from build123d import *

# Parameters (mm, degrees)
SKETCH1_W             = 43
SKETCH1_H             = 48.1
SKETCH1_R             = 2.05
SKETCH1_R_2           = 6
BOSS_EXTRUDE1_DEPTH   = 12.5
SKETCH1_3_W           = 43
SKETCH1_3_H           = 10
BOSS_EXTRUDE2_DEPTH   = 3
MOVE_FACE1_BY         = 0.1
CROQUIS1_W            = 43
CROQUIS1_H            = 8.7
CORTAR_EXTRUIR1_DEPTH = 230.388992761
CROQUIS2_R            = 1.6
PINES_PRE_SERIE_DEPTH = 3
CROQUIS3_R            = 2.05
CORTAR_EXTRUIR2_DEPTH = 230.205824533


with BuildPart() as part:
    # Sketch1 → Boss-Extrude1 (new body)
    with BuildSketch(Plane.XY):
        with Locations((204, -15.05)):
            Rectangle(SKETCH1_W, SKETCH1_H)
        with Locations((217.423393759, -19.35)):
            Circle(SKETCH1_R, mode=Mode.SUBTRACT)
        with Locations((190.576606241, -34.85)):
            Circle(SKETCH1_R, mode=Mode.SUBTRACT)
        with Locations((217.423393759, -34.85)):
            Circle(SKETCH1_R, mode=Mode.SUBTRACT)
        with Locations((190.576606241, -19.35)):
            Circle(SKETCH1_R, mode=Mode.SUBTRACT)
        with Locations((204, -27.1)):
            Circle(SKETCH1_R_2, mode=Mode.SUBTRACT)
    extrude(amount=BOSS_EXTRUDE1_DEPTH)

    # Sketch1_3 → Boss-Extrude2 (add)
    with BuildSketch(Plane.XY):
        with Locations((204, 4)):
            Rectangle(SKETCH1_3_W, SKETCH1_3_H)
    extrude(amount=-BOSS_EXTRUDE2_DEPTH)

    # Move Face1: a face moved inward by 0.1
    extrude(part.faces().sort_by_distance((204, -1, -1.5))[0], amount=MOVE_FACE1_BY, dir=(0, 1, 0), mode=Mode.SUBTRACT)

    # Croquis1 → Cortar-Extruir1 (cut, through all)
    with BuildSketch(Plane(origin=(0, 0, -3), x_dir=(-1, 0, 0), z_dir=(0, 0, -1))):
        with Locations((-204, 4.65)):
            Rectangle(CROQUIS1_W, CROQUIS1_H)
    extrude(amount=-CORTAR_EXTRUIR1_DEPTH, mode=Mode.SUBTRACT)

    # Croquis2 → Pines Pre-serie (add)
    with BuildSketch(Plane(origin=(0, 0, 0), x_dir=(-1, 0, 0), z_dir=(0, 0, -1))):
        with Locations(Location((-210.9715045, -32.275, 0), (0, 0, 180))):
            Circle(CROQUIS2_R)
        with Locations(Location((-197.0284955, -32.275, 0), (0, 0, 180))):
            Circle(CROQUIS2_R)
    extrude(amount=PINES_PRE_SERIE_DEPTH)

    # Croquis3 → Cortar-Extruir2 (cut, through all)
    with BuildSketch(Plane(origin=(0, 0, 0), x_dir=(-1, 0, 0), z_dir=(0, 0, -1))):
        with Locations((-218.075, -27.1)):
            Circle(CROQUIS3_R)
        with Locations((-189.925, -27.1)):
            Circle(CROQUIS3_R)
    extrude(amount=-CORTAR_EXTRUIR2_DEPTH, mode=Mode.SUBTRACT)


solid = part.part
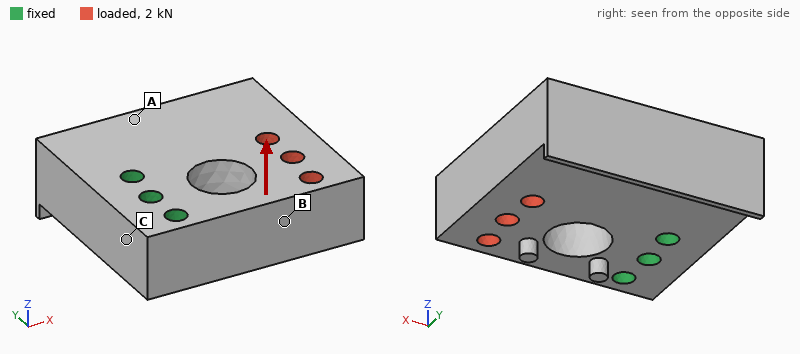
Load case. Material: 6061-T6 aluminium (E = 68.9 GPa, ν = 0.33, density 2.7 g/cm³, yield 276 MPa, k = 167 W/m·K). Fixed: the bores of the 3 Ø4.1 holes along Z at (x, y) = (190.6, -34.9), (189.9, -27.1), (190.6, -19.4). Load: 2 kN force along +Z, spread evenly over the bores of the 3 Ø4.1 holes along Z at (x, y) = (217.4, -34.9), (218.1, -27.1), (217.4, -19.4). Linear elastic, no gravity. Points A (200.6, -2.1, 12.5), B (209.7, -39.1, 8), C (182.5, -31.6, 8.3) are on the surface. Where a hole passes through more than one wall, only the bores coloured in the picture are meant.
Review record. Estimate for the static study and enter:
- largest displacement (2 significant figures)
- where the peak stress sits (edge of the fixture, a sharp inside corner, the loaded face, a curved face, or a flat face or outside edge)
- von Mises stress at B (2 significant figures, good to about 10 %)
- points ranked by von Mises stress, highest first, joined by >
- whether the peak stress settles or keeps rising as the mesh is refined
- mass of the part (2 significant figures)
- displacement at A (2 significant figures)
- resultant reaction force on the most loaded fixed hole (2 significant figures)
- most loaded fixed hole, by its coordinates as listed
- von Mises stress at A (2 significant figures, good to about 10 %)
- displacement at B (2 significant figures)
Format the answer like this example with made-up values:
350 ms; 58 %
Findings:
85 µm; edge of the fixture; 34 MPa; B > A > C; keeps rising; 51 g; 13 µm; 840 N; (190.6, -19.4); 22 MPa; 34 µm
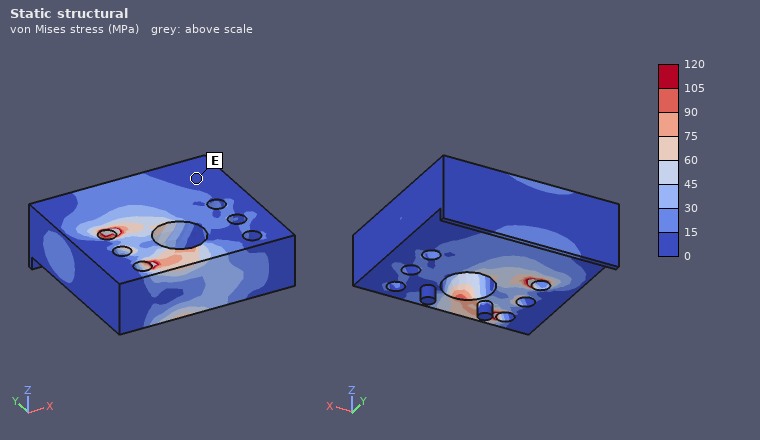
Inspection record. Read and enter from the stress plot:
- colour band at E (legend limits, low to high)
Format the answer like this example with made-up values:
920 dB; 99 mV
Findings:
0 to 15 MPa
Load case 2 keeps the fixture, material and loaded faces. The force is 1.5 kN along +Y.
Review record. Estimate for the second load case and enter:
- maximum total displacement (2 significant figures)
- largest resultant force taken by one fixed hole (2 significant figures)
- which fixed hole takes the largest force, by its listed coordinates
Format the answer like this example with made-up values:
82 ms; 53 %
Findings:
26 µm; 2.3 kN; (190.6, -19.4)
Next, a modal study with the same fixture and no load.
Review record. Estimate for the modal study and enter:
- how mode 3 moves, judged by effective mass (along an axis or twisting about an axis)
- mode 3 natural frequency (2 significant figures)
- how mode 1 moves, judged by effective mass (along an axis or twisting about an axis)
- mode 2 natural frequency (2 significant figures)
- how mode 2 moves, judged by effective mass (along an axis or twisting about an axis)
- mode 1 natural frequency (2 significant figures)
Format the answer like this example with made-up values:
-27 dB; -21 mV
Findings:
twisting about X; 11 kHz; along Z; 8400 Hz; along Y; 6200 Hz
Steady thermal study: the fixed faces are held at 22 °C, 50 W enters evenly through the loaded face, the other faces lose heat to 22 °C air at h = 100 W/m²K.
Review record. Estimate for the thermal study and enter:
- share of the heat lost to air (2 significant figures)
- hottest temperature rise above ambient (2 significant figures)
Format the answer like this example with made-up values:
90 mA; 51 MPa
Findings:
13 %; 27 K
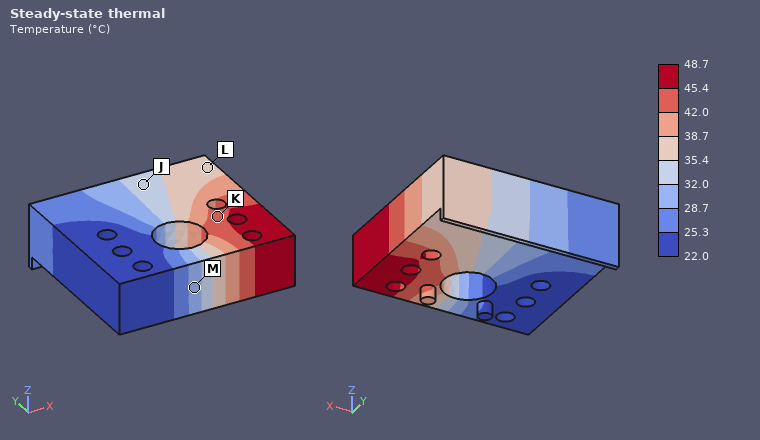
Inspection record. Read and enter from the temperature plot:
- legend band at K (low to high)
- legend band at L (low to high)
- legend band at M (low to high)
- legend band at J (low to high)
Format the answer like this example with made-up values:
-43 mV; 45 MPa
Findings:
42.0 to 45.4 °C; 35.4 to 38.7 °C; 28.7 to 32.0 °C; 32.0 to 35.4 °C
